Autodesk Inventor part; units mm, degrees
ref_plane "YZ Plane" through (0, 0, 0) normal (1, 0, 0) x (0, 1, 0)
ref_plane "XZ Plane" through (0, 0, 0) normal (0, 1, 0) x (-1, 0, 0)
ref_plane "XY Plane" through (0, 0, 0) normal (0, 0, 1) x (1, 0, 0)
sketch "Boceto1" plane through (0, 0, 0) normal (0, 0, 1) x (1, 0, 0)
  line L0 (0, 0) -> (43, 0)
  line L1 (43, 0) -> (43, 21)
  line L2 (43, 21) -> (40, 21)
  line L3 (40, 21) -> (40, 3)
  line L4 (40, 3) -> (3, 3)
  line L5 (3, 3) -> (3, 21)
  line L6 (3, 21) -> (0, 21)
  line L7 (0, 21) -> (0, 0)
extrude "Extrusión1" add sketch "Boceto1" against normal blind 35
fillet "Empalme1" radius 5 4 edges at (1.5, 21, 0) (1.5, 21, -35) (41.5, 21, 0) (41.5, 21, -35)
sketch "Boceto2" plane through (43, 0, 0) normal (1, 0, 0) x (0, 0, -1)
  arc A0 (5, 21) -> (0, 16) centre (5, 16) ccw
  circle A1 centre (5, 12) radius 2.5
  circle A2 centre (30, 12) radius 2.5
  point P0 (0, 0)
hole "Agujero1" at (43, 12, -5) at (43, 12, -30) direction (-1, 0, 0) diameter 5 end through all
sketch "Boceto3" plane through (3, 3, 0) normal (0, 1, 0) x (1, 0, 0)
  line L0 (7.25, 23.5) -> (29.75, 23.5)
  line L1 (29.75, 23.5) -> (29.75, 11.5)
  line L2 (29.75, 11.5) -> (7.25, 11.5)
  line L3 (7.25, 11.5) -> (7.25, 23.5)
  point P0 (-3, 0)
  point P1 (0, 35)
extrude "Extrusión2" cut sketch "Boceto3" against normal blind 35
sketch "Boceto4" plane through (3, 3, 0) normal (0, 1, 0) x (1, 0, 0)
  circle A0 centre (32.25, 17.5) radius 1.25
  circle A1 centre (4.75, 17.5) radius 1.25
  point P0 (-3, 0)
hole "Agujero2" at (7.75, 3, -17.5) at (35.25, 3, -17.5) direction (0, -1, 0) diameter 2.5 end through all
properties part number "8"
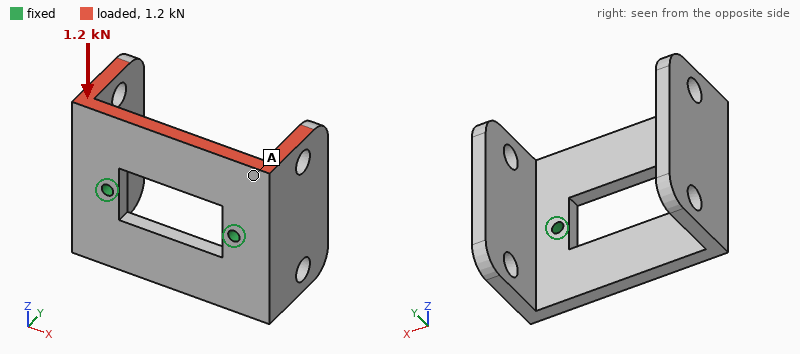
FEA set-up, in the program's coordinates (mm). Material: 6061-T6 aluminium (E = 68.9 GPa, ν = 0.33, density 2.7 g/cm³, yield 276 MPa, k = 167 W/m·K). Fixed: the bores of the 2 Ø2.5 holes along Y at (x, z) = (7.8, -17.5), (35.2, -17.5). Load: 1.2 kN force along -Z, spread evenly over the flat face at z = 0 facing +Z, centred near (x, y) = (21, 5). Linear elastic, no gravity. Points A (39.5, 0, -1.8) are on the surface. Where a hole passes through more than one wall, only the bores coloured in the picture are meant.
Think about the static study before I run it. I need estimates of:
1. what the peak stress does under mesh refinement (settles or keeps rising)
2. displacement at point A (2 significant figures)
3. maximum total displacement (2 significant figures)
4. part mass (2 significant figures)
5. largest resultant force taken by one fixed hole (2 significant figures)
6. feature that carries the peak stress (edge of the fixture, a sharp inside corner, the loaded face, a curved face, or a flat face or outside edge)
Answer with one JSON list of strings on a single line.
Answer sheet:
["keeps rising", "42 µm", "71 µm", "19 g", "610 N", "edge of the fixture"]
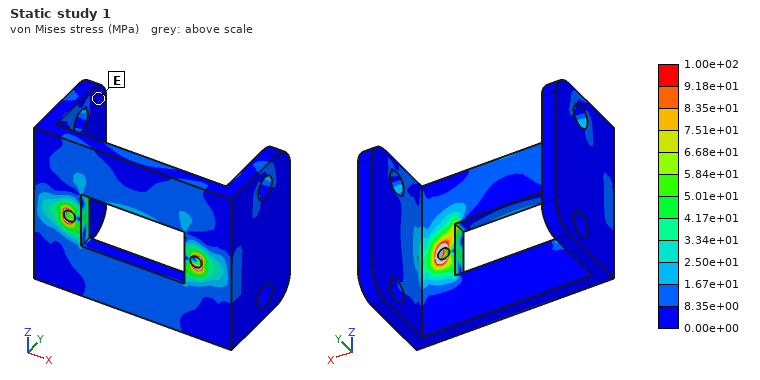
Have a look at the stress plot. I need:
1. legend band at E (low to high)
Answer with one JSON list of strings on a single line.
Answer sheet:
["0.00e+00 to 8.35e+00 MPa"]
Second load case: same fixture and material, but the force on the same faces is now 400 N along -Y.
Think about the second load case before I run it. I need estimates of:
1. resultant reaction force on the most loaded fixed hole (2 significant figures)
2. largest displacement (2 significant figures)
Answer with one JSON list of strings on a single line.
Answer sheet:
["210 N", "0.12 mm"]
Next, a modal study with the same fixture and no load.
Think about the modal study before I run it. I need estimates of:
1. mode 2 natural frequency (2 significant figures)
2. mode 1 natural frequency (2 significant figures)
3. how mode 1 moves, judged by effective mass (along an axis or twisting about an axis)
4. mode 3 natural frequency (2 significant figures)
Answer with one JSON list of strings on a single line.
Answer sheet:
["3700 Hz", "3300 Hz", "along Z", "4000 Hz"]
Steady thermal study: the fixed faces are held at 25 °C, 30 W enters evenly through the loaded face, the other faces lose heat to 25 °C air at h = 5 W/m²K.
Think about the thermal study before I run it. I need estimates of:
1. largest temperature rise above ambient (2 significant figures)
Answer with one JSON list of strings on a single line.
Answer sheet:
["32 K"]
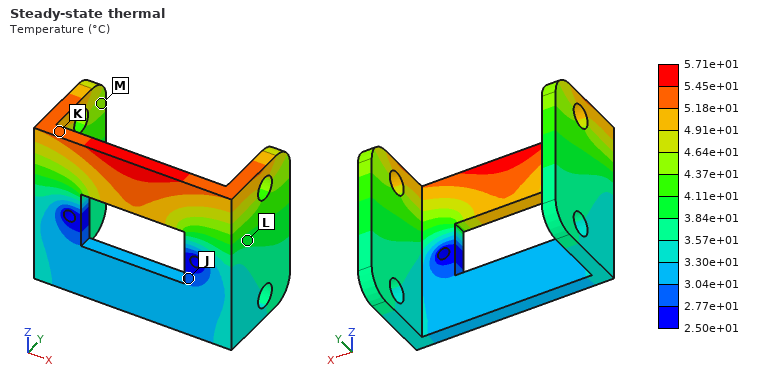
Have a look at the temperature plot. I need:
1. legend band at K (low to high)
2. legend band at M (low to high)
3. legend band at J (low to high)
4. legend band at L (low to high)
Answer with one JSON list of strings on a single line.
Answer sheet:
["5.18e+01 to 5.45e+01 °C", "4.37e+01 to 4.64e+01 °C", "2.77e+01 to 3.04e+01 °C", "3.84e+01 to 4.11e+01 °C"]
